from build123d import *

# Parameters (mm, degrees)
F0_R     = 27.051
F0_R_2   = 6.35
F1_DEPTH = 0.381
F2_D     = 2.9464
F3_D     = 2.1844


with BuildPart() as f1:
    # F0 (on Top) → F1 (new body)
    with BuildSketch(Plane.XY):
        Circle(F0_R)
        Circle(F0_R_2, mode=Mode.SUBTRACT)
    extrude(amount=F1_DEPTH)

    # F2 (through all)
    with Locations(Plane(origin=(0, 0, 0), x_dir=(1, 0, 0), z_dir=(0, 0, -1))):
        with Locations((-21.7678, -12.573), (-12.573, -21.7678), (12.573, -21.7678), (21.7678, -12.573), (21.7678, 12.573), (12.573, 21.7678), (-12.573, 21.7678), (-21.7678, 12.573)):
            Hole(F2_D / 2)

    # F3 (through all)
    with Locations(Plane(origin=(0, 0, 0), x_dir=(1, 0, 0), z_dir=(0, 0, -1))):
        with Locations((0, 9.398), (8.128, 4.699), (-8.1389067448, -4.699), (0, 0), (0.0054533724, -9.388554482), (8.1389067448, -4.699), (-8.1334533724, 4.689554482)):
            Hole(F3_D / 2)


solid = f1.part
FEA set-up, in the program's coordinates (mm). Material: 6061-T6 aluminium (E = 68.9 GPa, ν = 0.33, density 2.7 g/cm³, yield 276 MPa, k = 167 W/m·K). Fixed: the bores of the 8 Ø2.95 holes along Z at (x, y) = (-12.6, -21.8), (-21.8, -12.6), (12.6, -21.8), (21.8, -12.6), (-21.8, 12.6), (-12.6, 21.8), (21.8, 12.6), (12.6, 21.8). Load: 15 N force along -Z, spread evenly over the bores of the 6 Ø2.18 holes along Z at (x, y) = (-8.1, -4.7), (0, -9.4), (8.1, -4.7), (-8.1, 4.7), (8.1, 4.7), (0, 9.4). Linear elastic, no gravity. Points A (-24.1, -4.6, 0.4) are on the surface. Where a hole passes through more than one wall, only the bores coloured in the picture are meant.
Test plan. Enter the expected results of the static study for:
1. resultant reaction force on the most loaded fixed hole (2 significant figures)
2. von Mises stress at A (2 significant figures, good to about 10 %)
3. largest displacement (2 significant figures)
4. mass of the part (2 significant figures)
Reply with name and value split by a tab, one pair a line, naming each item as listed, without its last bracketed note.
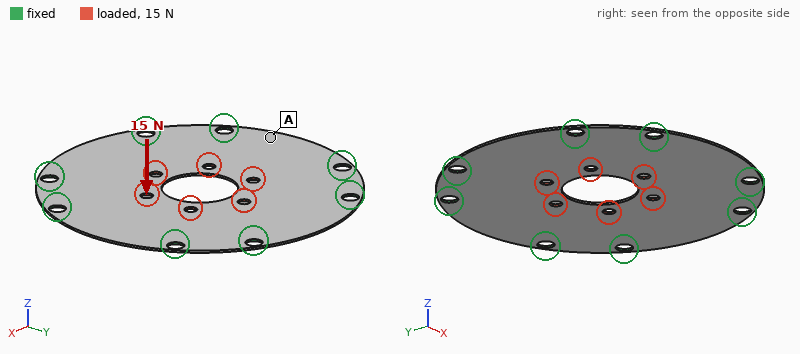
resultant reaction force on the most loaded fixed hole	1.9 N
von Mises stress at A	17 MPa
largest displacement	0.45 mm
mass of the part	2.2 g
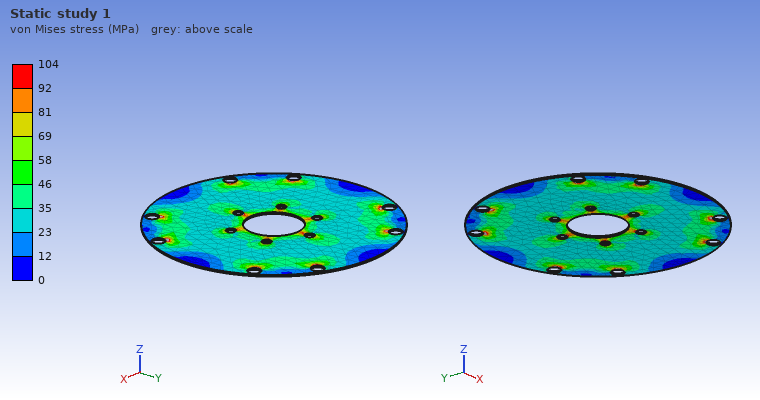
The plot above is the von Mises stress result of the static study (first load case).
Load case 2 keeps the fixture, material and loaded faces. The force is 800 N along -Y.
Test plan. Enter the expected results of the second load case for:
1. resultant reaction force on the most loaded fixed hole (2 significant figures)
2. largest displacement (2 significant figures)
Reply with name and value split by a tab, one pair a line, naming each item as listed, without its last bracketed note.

resultant reaction force on the most loaded fixed hole	140 N
largest displacement	13 µm
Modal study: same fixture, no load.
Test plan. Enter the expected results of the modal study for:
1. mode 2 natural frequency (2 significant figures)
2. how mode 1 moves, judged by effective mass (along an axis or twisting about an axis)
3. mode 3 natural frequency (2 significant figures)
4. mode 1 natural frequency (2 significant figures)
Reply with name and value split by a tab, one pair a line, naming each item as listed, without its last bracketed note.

mode 2 natural frequency	2700 Hz
how mode 1 moves, judged by effective mass	along Z
mode 3 natural frequency	2700 Hz
mode 1 natural frequency	1500 Hz
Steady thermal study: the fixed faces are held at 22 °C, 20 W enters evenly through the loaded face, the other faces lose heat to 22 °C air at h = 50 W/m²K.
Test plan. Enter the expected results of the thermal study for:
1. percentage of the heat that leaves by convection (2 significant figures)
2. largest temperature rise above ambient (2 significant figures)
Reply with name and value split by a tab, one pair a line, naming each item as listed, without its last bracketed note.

percentage of the heat that leaves by convection	22 %
largest temperature rise above ambient	58 K
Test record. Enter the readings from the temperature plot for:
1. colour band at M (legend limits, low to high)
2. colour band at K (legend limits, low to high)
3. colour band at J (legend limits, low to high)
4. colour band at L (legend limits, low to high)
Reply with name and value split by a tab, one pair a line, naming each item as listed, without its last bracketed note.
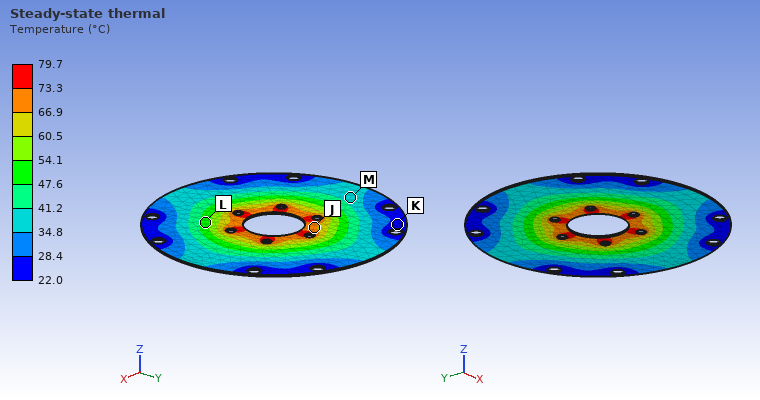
colour band at M	34.8 to 41.2 °C
colour band at K	22.0 to 28.4 °C
colour band at J	66.9 to 73.3 °C
colour band at L	47.6 to 54.1 °C
